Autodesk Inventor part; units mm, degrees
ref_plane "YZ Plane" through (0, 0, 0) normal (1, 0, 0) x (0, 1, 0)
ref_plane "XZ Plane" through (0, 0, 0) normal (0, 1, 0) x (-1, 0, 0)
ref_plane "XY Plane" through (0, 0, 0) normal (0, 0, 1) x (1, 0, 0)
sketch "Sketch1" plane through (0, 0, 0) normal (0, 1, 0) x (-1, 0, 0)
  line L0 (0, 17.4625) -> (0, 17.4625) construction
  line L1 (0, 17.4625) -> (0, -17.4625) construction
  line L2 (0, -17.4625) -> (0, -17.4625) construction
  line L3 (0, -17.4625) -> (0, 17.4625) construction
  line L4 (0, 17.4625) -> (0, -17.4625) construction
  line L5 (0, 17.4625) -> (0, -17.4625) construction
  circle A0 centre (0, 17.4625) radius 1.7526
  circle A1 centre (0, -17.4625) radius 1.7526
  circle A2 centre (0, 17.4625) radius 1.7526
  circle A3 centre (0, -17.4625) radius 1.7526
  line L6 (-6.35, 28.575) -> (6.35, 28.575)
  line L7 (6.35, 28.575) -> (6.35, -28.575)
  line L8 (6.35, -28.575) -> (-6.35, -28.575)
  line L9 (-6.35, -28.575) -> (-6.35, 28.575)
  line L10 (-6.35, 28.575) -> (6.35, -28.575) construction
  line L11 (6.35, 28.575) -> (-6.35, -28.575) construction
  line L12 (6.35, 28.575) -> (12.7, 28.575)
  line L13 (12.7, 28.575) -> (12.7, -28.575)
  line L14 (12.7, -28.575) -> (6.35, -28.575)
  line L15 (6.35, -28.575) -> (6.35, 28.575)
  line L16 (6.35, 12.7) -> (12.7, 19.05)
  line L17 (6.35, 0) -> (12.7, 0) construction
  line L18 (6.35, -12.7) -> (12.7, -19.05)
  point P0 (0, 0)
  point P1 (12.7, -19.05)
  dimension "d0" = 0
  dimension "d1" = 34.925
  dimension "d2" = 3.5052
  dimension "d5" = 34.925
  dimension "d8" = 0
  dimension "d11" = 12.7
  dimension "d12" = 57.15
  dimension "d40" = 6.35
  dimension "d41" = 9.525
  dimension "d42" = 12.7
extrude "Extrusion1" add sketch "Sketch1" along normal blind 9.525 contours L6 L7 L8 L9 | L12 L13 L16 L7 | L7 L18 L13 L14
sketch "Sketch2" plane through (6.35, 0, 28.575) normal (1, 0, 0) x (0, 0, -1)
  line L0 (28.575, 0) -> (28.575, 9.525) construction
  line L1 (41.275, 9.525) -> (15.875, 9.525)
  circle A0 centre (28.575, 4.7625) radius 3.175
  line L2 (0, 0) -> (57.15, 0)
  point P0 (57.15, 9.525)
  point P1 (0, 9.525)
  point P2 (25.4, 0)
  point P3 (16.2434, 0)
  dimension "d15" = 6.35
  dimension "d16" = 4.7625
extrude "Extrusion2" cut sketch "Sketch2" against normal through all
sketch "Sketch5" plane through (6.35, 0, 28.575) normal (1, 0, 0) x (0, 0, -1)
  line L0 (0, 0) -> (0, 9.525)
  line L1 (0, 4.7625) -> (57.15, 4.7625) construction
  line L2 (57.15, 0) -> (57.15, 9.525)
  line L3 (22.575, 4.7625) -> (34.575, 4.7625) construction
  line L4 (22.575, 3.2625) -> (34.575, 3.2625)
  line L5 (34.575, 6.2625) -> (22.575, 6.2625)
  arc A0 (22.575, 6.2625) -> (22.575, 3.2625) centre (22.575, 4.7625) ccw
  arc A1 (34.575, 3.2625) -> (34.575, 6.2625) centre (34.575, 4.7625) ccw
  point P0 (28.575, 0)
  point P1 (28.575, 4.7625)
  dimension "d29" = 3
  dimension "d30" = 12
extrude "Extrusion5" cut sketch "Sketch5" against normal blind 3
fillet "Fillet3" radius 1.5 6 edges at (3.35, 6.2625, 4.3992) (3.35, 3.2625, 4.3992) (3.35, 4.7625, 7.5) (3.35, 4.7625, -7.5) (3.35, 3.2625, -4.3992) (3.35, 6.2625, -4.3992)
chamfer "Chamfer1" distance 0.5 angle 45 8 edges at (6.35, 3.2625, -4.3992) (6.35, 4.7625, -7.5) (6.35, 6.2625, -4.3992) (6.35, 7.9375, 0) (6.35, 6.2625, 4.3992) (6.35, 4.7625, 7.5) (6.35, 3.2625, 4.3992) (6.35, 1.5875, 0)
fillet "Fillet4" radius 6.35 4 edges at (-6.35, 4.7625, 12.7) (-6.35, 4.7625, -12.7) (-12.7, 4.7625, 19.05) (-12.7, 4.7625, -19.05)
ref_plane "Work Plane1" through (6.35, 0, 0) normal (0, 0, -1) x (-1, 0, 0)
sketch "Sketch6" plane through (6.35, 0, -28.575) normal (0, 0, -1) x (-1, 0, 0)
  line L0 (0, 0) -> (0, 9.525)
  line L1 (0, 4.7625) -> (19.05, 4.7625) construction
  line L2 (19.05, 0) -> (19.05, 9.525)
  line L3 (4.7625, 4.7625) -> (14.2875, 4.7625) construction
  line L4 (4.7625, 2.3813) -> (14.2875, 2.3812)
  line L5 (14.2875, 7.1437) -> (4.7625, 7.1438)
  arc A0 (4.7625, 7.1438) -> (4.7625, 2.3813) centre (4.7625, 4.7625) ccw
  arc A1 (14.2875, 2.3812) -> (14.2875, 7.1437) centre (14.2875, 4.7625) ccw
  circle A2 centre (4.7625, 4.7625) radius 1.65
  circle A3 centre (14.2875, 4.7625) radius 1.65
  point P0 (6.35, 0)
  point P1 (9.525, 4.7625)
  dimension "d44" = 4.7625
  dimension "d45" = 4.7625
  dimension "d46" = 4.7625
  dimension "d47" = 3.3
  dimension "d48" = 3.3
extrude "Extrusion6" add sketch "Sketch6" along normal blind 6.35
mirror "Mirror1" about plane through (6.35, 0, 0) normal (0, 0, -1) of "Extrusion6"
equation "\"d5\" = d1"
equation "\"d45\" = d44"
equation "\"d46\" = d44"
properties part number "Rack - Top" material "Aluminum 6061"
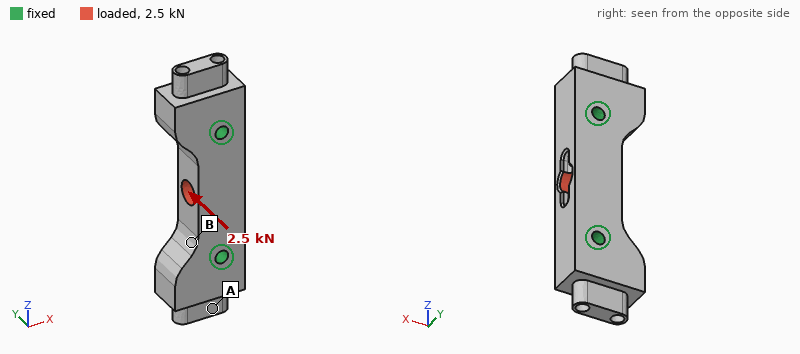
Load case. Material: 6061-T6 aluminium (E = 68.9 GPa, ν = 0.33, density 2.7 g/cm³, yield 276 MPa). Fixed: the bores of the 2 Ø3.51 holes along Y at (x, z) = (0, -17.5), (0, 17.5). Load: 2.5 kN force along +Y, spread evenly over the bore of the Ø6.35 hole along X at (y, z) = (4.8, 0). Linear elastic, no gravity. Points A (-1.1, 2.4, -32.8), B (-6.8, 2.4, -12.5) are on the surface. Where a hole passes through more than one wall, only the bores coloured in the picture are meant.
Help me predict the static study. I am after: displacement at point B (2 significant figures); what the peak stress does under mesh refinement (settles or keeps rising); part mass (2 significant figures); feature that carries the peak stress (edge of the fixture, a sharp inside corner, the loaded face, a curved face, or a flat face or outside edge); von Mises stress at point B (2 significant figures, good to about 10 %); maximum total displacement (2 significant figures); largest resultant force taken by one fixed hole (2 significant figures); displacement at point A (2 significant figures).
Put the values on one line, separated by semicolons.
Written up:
4.5 µm; keeps rising; 23 g; edge of the fixture; 19 MPa; 19 µm; 1.3 kN; 3.3 µm
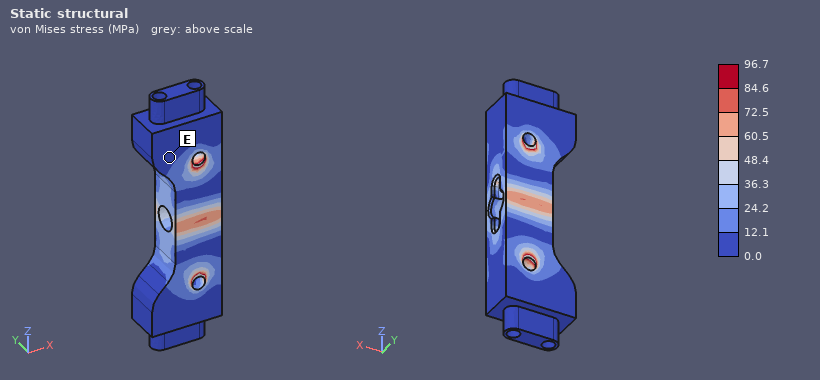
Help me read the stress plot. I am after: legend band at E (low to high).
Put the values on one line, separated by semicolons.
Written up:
0.0 to 12.1 MPa
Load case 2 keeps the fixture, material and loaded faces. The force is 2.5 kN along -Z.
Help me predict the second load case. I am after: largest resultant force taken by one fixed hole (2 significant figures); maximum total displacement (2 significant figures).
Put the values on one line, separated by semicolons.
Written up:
1.3 kN; 3.0 µm
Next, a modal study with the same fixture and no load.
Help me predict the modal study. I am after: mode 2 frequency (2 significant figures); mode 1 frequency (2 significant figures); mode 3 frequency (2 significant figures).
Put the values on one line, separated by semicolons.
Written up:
24 kHz; 18 kHz; 24 kHz
